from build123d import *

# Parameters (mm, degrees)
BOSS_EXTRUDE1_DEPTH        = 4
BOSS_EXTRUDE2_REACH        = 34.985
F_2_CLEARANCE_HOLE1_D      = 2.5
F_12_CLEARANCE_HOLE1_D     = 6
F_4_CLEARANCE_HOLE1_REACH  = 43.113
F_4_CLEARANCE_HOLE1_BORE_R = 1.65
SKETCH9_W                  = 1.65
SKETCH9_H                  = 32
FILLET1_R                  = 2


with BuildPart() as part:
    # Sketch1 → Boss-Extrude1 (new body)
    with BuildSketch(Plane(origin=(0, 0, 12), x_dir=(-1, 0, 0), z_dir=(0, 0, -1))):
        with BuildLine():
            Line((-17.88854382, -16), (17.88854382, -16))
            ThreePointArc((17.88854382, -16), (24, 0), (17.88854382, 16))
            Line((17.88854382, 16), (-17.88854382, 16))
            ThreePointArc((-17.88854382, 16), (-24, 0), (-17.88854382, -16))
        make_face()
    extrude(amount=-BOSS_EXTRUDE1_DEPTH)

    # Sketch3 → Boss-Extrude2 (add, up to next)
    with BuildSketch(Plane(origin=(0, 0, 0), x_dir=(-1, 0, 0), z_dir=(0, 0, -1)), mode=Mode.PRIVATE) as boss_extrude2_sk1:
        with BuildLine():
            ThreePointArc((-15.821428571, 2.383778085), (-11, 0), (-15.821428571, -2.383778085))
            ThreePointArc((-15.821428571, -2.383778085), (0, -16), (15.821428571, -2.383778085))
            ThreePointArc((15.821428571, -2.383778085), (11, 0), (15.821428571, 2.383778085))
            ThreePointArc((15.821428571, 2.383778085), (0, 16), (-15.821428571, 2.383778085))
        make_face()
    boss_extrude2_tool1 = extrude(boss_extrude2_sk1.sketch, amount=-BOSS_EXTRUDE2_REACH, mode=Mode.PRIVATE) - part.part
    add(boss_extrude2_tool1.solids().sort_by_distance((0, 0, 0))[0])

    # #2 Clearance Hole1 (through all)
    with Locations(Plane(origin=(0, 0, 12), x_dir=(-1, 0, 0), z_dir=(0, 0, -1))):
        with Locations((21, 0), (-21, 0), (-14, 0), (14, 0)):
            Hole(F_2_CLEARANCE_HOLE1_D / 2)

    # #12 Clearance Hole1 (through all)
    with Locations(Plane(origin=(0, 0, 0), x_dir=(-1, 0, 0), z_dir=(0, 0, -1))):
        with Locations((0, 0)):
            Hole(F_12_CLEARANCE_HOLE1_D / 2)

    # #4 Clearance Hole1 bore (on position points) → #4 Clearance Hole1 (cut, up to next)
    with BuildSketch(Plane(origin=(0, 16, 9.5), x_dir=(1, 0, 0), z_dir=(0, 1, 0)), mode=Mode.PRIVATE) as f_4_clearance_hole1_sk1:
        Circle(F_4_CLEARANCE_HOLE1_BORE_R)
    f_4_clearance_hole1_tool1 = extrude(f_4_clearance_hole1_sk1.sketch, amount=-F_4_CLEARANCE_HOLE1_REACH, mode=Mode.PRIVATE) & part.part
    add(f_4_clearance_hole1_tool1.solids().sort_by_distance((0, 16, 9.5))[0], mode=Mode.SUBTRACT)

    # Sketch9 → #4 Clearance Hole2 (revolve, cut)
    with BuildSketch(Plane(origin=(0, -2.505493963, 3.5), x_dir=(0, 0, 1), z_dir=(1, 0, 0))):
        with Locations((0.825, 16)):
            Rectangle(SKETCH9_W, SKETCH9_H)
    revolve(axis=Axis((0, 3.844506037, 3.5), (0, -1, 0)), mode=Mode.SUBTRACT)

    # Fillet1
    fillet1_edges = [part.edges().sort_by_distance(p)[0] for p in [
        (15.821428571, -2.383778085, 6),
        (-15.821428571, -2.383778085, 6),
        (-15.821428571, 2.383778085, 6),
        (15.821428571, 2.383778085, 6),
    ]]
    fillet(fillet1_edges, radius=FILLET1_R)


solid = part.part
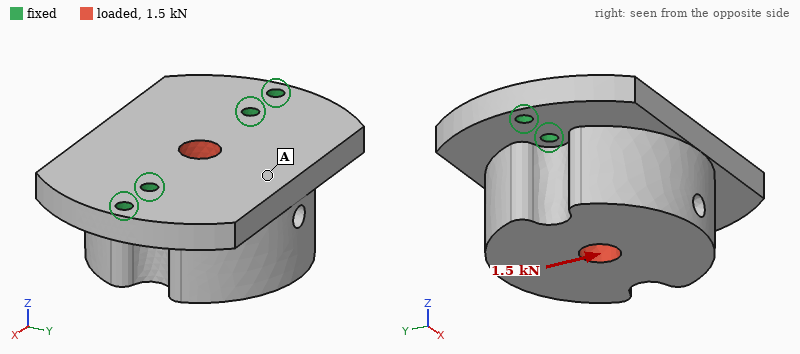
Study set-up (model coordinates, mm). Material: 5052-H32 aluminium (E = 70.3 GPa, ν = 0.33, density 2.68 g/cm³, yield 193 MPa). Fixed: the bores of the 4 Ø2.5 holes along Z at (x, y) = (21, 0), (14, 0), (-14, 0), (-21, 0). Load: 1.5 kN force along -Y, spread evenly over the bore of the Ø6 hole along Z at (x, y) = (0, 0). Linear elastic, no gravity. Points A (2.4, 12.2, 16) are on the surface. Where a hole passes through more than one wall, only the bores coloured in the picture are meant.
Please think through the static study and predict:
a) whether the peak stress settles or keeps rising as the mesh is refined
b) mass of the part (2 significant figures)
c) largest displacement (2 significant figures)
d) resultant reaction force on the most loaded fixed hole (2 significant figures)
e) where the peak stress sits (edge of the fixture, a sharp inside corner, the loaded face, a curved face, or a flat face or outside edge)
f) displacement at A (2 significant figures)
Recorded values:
keeps rising
37 g
35 µm
710 N
edge of the fixture
19 µm
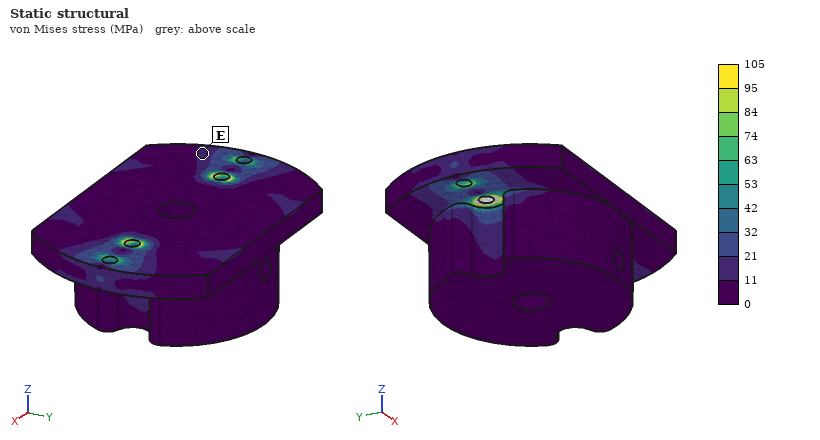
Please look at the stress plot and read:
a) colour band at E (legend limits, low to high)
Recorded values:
11 to 21 MPa
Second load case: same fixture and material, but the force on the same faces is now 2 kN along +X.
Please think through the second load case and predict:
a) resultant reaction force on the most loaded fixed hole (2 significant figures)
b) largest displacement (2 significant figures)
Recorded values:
830 N
4.5 µm
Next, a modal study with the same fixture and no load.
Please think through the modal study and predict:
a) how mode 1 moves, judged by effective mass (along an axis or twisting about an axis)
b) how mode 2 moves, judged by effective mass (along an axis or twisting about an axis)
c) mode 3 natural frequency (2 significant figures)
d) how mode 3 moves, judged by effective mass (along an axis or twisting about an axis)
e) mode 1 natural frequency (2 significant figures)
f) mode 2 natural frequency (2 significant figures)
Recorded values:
along Y
along Z
21 kHz
along X
5700 Hz
17 kHz
